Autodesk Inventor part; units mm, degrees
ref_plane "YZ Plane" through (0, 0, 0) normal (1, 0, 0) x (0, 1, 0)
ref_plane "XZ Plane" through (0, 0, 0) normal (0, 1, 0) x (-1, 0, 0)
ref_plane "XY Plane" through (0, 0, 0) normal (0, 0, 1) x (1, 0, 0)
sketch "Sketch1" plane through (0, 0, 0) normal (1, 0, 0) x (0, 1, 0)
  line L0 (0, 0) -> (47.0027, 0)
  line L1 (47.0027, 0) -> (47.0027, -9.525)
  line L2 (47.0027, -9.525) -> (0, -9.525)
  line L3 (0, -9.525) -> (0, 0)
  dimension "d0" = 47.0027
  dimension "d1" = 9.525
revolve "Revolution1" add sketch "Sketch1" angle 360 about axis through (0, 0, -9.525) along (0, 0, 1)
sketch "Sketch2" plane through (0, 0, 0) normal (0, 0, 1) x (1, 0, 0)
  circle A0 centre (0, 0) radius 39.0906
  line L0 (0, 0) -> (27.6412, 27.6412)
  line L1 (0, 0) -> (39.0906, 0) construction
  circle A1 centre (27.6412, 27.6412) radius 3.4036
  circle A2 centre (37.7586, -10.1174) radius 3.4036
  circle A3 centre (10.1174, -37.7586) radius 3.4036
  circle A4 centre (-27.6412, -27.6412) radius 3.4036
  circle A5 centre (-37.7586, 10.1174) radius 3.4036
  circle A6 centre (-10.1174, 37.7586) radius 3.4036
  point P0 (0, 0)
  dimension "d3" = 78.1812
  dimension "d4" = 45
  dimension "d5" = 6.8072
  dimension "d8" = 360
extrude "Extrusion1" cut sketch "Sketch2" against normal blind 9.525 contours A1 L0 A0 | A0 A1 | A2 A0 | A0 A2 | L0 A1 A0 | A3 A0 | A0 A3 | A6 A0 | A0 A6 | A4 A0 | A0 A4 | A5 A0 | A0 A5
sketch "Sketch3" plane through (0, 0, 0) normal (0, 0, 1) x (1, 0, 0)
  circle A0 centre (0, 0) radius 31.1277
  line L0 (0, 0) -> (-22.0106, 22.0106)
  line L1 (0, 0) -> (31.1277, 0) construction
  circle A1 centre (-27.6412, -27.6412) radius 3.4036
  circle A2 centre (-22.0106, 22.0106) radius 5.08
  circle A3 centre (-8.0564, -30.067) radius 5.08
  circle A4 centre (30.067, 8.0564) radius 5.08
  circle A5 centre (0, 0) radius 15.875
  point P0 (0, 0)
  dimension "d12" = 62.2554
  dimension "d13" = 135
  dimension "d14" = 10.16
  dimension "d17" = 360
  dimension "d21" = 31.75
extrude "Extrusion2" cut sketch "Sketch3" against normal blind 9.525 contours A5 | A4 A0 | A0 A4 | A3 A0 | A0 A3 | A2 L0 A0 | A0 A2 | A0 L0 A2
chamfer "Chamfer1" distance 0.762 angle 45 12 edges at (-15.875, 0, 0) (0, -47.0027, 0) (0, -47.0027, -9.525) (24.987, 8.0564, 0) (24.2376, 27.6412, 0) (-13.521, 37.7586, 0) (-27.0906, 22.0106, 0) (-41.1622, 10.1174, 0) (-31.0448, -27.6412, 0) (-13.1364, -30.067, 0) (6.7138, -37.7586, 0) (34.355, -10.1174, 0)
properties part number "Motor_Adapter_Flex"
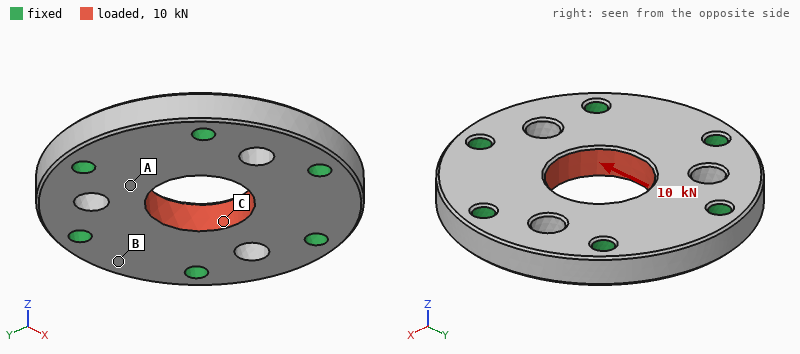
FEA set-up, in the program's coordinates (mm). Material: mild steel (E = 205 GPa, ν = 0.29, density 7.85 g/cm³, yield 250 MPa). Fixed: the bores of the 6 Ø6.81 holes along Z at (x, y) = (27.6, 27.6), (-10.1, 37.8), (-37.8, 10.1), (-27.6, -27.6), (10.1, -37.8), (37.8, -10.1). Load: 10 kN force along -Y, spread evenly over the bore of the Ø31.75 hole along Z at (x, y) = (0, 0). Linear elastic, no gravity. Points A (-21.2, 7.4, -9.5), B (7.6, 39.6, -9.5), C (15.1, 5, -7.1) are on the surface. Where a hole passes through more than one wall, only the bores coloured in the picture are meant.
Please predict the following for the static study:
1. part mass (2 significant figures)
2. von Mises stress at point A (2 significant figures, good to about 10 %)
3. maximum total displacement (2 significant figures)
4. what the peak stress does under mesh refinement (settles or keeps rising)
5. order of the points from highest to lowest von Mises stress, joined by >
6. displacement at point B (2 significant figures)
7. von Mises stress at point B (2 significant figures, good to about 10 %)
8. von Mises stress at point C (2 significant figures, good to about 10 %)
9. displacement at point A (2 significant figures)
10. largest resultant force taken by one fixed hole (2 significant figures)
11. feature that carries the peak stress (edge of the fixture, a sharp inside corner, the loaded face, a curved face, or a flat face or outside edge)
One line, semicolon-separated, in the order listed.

420 g; 7.6 MPa; 1.8 µm; keeps rising; C > A > B; 0.82 µm; 3.3 MPa; 20 MPa; 1.0 µm; 2.4 kN; edge of the fixture
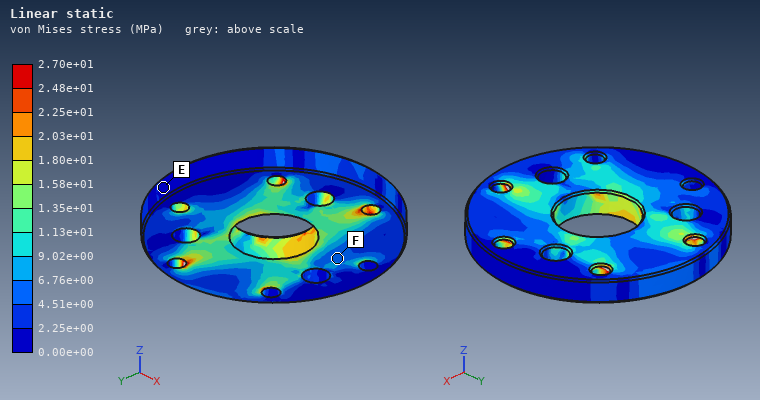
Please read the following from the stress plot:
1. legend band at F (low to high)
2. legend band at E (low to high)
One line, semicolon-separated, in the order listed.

4.51e+00 to 6.76e+00 MPa; 0.00e+00 to 2.25e+00 MPa
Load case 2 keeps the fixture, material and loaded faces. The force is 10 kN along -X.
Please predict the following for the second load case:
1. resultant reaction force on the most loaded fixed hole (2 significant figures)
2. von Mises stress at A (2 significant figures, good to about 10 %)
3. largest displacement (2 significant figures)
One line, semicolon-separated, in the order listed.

2.4 kN; 13 MPa; 1.8 µm
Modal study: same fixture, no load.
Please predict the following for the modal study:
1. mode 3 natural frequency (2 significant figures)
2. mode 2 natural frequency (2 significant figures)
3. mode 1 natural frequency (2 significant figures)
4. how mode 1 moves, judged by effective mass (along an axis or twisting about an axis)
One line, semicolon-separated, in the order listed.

20 kHz; 20 kHz; 15 kHz; along Z
